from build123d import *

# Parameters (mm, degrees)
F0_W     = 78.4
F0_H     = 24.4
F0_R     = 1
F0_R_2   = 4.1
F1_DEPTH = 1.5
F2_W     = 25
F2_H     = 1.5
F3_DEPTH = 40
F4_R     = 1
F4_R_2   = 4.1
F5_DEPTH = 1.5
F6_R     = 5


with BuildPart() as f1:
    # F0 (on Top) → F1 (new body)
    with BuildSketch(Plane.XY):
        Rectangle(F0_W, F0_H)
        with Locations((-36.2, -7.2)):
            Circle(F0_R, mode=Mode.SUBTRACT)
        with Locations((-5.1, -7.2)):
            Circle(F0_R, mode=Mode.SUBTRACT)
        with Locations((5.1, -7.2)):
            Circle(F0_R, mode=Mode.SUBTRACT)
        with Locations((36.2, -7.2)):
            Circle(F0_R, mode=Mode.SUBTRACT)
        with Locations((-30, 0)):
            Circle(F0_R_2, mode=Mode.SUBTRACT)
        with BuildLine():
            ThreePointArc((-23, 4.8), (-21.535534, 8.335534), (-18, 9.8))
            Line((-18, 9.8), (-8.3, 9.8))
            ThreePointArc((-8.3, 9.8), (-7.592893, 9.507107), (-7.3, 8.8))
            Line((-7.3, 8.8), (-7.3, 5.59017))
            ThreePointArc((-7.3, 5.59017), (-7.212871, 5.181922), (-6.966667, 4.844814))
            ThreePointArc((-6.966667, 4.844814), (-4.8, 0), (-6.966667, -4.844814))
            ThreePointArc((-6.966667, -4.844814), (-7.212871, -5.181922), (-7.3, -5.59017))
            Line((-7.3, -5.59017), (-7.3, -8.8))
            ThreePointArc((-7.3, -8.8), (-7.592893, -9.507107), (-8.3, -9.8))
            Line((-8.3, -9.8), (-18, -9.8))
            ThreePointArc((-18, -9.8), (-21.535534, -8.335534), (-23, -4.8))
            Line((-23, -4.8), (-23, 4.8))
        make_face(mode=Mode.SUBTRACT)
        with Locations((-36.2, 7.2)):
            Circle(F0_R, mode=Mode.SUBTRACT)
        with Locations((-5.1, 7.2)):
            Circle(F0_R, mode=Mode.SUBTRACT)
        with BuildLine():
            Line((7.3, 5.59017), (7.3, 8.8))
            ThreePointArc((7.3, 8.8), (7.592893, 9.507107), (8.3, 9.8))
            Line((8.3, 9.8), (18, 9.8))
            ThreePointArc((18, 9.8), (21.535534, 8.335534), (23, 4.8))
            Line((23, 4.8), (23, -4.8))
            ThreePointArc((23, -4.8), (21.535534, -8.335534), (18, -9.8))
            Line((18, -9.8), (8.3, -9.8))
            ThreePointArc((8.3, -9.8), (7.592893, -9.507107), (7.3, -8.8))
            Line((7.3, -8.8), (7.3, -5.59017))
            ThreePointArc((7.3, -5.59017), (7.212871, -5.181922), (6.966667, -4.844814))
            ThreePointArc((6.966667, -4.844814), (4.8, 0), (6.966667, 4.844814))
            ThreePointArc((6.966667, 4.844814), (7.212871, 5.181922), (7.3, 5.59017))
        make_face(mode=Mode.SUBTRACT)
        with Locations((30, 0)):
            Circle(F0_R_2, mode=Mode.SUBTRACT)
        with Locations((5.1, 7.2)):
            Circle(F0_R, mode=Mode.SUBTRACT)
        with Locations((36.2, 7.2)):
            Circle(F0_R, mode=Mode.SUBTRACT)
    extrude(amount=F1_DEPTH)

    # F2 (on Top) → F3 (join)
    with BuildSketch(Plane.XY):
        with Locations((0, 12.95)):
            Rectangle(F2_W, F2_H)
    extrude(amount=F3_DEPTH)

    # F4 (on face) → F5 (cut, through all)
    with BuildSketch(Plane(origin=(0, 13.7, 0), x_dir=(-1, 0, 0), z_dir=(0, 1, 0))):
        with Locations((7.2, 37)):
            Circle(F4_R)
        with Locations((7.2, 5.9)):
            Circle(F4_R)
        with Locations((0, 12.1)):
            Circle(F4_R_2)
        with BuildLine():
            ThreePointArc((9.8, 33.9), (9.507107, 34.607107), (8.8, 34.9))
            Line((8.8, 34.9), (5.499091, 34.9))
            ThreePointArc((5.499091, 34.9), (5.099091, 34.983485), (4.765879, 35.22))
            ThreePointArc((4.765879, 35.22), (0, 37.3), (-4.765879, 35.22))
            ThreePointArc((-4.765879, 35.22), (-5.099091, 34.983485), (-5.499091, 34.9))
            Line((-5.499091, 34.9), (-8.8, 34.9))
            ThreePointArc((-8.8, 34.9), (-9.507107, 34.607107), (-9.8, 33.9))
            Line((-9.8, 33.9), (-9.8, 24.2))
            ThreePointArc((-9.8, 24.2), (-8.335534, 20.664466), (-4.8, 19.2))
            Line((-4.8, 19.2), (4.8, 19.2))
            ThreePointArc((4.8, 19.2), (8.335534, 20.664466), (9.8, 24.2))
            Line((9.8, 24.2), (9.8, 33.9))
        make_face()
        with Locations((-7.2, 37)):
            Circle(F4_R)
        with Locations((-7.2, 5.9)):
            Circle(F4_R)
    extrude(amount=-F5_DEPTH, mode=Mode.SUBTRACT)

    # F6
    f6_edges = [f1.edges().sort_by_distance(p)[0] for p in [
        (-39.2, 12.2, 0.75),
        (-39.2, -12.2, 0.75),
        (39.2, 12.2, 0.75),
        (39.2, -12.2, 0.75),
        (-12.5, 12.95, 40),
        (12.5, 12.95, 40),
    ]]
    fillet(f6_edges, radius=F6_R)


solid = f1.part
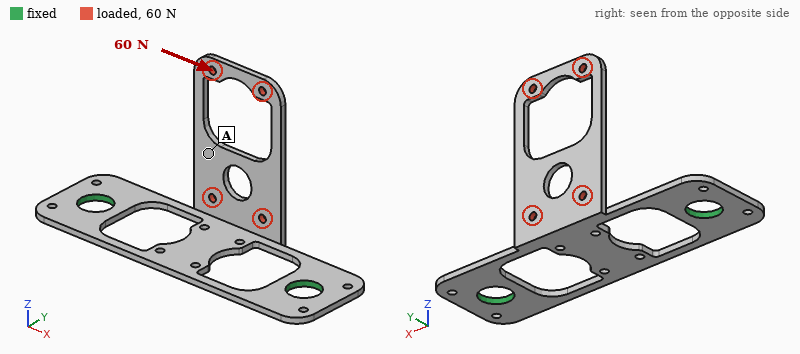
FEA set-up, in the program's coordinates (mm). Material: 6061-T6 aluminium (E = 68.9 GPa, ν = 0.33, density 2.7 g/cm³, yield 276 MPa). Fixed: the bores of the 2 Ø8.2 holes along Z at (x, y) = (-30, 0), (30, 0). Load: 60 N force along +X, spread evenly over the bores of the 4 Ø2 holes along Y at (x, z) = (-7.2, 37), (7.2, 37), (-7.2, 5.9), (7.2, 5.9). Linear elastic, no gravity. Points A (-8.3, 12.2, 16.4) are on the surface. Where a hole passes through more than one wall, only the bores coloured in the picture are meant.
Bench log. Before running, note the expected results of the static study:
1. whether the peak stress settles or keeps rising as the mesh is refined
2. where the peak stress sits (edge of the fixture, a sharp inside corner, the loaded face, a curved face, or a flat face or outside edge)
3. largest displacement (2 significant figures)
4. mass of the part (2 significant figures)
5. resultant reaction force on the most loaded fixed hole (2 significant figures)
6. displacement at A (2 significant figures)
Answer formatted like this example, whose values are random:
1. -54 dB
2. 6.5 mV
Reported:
1. keeps rising
2. a sharp inside corner
3. 0.50 mm
4. 7.1 g
5. 45 N
6. 0.21 mm
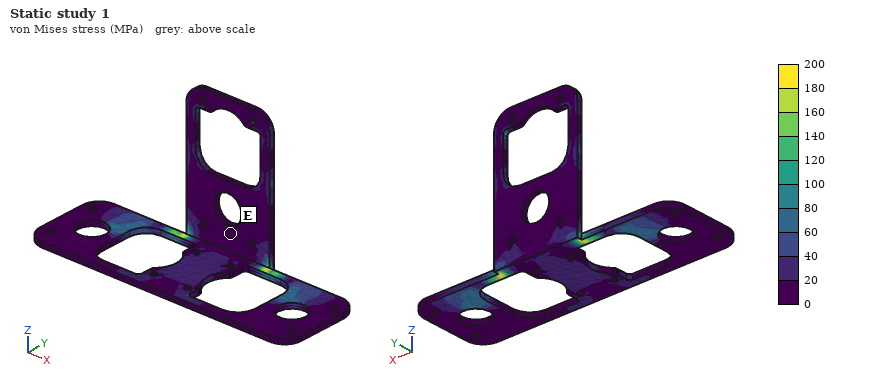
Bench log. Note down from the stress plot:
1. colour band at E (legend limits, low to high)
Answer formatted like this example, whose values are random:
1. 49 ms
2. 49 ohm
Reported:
1. 0 to 20 MPa
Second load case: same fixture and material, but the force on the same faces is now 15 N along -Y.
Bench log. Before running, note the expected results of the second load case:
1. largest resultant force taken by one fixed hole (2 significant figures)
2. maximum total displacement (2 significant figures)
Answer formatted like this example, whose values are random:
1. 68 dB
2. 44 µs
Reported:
1. 9.0 N
2. 1.0 mm
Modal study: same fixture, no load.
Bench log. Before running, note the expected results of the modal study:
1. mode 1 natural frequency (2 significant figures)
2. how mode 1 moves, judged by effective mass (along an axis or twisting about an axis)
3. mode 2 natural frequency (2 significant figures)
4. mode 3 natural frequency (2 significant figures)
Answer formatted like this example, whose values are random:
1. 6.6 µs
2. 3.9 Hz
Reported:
1. 590 Hz
2. along Y
3. 1500 Hz
4. 1500 Hz
